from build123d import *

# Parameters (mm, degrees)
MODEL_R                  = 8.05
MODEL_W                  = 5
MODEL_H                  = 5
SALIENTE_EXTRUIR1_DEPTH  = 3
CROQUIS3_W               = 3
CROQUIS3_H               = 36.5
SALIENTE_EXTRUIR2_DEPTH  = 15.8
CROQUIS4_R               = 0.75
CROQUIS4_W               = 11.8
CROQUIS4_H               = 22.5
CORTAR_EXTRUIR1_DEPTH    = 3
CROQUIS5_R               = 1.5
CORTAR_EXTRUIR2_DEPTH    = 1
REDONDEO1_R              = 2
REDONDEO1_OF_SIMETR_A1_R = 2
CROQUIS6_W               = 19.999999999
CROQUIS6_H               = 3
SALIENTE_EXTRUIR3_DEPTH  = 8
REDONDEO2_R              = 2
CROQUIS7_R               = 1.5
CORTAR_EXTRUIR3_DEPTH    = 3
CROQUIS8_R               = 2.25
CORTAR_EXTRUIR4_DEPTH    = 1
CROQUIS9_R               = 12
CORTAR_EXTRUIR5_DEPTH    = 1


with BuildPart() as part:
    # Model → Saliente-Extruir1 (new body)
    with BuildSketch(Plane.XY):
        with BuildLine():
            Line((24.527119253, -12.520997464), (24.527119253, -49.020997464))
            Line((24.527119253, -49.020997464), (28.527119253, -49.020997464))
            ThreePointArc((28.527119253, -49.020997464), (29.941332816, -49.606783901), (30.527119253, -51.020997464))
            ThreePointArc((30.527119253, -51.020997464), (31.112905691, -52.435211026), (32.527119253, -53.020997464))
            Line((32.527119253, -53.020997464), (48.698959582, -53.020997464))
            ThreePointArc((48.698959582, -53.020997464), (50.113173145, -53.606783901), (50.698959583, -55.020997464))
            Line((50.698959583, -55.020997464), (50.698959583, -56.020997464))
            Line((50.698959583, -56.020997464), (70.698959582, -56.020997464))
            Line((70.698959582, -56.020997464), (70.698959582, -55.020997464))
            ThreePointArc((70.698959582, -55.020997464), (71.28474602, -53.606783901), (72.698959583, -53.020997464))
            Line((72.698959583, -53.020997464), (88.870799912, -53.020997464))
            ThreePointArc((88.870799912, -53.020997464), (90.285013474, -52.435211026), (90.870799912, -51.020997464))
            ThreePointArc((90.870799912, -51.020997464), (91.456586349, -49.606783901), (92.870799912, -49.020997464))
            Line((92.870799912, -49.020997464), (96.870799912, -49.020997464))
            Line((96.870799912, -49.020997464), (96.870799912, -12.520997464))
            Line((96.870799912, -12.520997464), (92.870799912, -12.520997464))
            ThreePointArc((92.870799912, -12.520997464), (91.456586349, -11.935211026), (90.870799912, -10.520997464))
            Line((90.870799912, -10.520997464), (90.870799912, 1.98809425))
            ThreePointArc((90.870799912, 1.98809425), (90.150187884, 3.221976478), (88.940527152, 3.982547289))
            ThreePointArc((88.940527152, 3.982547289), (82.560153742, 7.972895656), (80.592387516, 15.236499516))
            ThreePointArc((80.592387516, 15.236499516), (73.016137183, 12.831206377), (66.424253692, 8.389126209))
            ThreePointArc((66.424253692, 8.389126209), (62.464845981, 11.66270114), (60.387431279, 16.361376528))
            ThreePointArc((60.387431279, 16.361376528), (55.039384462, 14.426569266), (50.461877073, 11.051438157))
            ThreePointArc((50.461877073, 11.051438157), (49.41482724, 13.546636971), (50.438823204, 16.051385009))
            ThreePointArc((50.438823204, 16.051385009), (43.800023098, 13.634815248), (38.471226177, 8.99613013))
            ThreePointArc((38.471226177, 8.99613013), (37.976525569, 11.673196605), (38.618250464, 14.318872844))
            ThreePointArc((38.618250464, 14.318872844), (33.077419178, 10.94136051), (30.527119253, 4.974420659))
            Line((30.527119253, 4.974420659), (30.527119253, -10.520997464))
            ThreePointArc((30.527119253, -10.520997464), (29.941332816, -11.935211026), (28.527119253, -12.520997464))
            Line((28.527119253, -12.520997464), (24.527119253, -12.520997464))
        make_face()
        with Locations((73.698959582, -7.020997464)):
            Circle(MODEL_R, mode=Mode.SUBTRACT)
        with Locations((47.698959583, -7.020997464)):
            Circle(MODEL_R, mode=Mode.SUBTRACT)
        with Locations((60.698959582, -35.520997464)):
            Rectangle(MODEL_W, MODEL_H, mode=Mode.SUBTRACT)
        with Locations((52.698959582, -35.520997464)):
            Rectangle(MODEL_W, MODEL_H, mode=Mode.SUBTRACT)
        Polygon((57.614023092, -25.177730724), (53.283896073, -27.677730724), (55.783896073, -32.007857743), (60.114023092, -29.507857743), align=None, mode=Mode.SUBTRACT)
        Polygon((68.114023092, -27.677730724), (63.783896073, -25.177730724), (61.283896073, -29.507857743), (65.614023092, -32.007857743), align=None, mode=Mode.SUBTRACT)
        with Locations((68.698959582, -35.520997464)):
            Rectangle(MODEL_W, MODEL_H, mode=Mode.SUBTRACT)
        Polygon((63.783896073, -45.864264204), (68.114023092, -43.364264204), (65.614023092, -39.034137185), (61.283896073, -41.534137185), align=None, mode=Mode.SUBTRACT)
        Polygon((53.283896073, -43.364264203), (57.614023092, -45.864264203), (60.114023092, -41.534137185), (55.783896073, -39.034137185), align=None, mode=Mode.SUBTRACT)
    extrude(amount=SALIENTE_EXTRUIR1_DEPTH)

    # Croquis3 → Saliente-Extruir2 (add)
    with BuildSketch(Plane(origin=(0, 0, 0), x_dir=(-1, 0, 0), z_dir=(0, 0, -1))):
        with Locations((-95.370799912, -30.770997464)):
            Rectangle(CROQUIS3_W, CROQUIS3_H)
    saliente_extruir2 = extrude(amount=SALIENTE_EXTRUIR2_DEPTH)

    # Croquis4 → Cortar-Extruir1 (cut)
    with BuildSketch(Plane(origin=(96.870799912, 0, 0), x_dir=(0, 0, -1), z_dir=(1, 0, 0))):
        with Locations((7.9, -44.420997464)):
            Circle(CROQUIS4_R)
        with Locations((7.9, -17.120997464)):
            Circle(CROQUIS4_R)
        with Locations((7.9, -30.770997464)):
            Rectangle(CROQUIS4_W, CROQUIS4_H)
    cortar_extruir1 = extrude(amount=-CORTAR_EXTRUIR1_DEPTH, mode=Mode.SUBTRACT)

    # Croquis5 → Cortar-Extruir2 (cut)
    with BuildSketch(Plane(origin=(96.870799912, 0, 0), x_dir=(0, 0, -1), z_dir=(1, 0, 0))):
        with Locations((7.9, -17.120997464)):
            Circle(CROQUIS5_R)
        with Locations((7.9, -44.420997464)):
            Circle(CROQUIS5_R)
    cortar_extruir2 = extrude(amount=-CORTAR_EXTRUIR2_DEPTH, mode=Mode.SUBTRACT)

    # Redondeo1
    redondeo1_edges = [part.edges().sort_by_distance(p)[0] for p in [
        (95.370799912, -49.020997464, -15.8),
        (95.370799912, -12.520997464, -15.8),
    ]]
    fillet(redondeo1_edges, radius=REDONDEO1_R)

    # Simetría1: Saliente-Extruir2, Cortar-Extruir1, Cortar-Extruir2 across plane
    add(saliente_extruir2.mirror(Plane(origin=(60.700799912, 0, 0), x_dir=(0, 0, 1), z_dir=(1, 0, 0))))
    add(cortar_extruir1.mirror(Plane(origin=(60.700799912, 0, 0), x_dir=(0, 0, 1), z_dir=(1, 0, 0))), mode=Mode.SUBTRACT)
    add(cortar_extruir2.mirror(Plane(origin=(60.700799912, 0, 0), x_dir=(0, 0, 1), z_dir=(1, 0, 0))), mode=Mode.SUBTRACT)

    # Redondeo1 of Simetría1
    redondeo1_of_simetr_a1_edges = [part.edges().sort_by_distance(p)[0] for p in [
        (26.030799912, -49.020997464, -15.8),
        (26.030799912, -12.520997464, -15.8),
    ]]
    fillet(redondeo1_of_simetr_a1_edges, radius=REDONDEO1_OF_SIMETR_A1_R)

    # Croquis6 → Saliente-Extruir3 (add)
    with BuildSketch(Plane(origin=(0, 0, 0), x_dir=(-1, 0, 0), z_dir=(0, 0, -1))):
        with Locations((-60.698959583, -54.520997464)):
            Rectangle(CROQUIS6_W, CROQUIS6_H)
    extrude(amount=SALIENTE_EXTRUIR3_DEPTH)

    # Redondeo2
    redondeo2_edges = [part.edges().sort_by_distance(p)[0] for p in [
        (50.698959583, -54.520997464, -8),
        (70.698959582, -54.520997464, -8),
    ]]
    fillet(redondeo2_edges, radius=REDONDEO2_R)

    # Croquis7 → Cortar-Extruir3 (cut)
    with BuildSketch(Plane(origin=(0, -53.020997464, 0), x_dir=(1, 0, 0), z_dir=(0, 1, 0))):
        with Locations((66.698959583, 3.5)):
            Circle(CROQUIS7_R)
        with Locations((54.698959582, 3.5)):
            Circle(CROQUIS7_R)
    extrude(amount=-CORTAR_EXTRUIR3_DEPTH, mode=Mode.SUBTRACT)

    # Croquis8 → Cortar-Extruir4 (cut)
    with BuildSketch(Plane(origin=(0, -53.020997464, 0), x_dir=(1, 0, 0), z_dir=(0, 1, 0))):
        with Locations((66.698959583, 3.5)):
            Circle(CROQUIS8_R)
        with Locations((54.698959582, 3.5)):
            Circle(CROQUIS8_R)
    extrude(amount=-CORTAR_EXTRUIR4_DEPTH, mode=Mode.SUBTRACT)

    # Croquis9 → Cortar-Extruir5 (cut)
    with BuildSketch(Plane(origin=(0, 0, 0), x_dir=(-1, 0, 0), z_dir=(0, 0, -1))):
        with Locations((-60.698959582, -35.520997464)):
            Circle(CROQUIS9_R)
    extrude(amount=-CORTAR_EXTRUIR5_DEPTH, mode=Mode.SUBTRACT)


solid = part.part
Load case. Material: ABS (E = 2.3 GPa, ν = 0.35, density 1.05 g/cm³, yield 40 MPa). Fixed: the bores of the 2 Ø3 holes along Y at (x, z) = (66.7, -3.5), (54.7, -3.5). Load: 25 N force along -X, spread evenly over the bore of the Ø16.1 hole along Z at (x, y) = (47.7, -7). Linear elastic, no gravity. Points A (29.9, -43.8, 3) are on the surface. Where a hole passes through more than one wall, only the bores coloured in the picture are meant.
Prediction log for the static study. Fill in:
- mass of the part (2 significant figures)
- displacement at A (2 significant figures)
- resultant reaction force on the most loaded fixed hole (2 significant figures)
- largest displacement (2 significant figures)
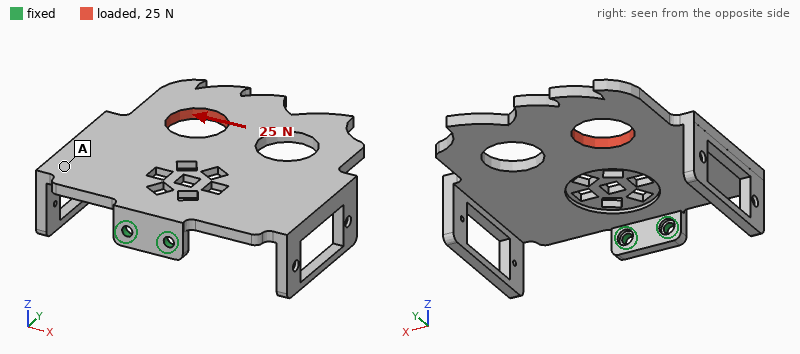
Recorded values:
14 g
0.51 mm
90 N
1.0 mm
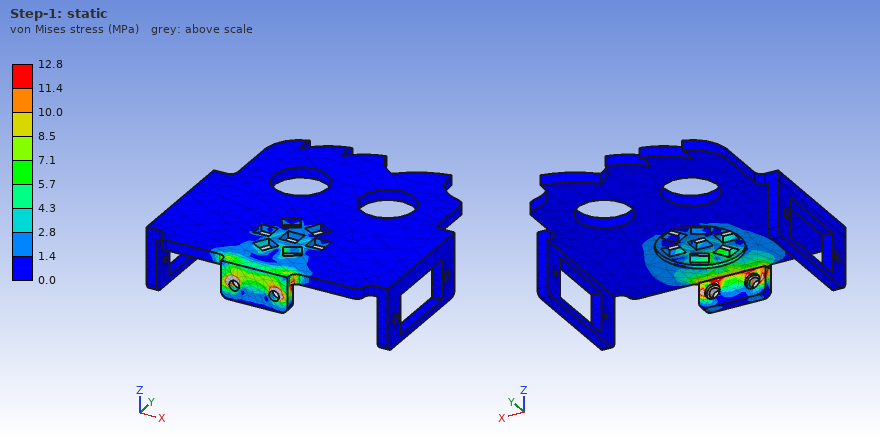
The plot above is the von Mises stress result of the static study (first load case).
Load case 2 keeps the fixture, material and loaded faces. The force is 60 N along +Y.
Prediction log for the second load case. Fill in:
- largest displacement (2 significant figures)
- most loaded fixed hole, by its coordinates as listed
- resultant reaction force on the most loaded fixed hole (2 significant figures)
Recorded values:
1.1 mm
(54.7, -3.5)
87 N
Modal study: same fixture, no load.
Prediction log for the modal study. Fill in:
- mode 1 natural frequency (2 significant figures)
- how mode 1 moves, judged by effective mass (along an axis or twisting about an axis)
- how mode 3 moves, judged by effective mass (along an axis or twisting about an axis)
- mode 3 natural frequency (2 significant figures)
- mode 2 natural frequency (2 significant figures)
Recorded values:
97 Hz
along Z
along X
330 Hz
190 Hz
